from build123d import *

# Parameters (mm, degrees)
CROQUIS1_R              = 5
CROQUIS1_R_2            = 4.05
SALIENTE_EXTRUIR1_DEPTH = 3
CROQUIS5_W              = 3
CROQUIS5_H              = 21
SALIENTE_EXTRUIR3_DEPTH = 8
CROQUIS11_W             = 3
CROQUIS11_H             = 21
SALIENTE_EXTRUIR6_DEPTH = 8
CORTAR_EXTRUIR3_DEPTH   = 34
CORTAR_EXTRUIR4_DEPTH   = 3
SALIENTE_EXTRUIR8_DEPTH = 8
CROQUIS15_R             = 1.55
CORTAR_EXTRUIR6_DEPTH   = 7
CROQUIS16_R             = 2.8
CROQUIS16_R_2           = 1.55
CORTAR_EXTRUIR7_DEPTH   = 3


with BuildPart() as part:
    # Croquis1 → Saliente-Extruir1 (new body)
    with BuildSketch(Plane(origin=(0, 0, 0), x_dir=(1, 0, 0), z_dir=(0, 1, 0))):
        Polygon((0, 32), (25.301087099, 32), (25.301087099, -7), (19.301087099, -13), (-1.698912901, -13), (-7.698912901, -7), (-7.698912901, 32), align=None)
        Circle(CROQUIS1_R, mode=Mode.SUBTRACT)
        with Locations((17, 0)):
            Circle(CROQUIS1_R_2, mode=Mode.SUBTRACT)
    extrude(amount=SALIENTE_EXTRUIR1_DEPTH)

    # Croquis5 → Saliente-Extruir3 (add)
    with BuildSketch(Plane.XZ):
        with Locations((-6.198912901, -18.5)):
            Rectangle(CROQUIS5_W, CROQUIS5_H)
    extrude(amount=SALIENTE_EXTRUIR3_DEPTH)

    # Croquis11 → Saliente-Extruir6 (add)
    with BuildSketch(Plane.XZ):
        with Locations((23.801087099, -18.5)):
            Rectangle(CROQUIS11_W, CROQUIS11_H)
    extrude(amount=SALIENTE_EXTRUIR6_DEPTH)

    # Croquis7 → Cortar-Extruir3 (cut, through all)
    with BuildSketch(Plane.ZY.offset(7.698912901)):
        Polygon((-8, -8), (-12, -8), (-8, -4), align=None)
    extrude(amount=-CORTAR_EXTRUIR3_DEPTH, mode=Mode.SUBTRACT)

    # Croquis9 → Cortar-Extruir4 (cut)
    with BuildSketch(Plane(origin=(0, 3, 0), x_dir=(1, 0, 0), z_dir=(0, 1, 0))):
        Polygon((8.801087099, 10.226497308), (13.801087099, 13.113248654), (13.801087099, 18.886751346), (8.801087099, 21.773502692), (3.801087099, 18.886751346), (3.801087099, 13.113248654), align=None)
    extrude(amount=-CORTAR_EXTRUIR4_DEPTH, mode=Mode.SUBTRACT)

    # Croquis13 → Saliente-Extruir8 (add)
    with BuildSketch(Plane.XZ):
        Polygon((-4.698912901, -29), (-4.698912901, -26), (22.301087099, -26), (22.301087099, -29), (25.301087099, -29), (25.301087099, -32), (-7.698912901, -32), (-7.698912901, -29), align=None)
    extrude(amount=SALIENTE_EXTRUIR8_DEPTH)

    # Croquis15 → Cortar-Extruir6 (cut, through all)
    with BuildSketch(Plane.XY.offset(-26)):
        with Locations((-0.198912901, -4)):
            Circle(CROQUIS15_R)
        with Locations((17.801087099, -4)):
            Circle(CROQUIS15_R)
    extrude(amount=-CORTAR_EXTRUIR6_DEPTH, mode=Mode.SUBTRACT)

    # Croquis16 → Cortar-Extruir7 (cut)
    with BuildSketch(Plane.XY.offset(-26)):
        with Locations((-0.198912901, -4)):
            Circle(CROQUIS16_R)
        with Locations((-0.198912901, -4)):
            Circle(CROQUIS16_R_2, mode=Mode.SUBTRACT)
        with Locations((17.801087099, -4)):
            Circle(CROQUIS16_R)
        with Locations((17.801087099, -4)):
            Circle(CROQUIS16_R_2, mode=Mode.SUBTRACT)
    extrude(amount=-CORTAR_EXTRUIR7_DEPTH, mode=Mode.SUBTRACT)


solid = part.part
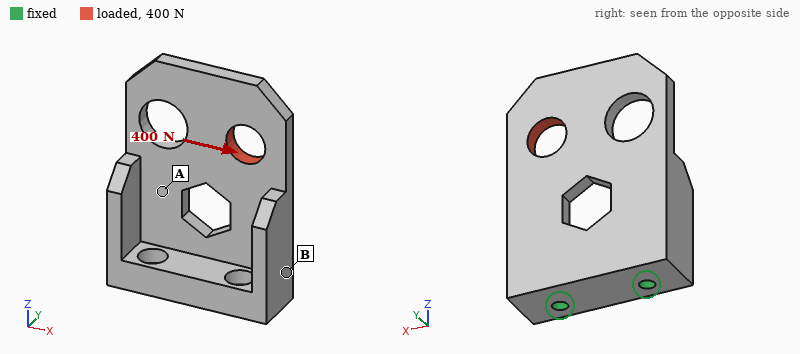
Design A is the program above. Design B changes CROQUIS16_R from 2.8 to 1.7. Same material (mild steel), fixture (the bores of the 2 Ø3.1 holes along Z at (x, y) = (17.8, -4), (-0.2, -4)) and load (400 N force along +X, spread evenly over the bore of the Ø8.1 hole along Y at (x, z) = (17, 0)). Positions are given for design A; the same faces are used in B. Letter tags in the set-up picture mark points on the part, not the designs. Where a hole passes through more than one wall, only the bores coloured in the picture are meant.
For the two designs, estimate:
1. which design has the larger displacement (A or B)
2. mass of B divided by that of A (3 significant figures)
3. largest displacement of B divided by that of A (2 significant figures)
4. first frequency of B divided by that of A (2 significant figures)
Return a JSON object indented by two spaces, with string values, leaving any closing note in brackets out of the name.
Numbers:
{
  "which design has the larger displacement": "A",
  "mass of B divided by that of A": "1.02",
  "largest displacement of B divided by that of A": "0.90",
  "first frequency of B divided by that of A": "1.0"
}
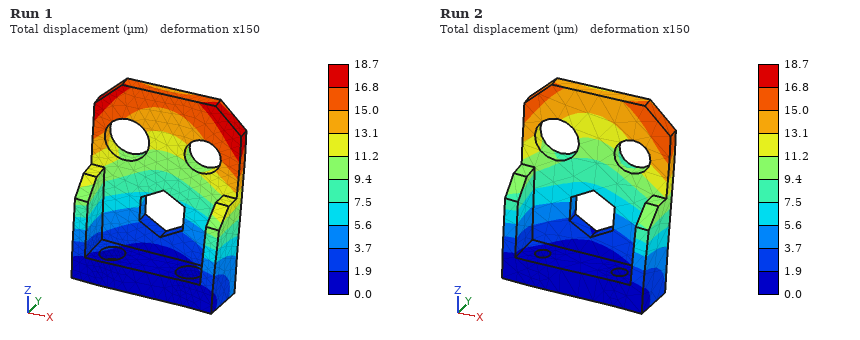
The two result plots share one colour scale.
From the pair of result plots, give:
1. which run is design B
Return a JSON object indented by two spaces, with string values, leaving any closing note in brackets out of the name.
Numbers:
{
  "which run is design B": "Run 2"
}
